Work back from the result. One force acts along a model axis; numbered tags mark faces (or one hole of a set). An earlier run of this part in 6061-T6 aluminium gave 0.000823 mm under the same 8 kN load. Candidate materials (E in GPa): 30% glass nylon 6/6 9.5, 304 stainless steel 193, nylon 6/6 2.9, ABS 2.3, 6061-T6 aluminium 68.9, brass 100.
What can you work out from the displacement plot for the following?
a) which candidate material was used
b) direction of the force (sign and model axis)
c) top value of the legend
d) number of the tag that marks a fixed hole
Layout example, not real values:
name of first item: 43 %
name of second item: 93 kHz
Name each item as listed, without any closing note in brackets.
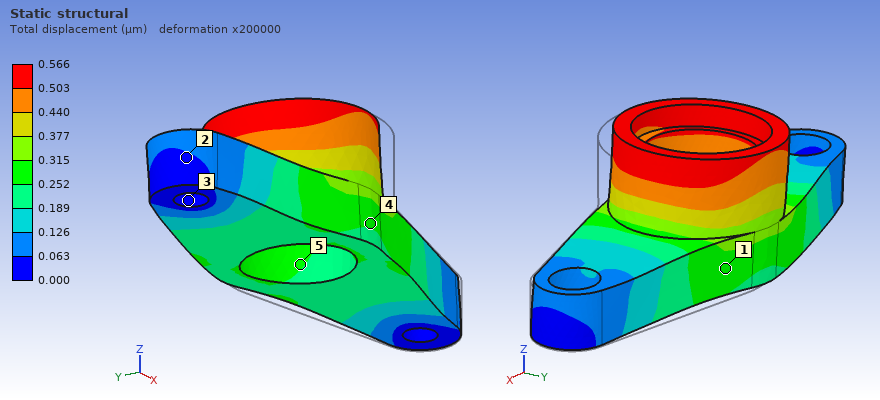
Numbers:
which candidate material was used: brass
direction of the force: -X
top value of the legend: 0.566 µm
number of the tag that marks a fixed hole: 3
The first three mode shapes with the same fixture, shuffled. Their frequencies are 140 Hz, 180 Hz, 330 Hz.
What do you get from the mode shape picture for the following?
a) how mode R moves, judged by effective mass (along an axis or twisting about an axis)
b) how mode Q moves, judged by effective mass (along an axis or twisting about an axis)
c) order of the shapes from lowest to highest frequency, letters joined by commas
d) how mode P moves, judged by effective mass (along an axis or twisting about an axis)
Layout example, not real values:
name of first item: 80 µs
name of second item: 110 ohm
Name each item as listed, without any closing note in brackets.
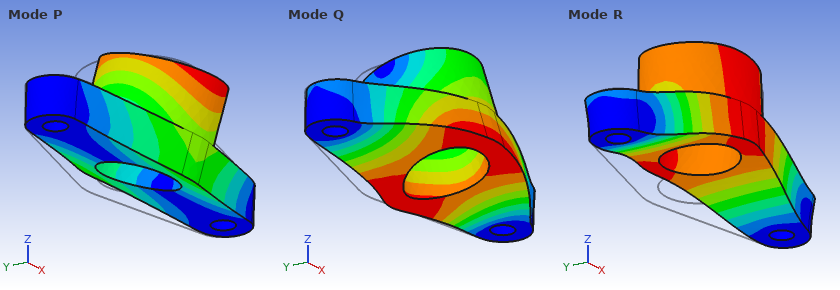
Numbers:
how mode R moves, judged by effective mass: along Z
how mode Q moves, judged by effective mass: along Y
order of the shapes from lowest to highest frequency, letters joined by commas: P, R, Q
how mode P moves, judged by effective mass: along Y
